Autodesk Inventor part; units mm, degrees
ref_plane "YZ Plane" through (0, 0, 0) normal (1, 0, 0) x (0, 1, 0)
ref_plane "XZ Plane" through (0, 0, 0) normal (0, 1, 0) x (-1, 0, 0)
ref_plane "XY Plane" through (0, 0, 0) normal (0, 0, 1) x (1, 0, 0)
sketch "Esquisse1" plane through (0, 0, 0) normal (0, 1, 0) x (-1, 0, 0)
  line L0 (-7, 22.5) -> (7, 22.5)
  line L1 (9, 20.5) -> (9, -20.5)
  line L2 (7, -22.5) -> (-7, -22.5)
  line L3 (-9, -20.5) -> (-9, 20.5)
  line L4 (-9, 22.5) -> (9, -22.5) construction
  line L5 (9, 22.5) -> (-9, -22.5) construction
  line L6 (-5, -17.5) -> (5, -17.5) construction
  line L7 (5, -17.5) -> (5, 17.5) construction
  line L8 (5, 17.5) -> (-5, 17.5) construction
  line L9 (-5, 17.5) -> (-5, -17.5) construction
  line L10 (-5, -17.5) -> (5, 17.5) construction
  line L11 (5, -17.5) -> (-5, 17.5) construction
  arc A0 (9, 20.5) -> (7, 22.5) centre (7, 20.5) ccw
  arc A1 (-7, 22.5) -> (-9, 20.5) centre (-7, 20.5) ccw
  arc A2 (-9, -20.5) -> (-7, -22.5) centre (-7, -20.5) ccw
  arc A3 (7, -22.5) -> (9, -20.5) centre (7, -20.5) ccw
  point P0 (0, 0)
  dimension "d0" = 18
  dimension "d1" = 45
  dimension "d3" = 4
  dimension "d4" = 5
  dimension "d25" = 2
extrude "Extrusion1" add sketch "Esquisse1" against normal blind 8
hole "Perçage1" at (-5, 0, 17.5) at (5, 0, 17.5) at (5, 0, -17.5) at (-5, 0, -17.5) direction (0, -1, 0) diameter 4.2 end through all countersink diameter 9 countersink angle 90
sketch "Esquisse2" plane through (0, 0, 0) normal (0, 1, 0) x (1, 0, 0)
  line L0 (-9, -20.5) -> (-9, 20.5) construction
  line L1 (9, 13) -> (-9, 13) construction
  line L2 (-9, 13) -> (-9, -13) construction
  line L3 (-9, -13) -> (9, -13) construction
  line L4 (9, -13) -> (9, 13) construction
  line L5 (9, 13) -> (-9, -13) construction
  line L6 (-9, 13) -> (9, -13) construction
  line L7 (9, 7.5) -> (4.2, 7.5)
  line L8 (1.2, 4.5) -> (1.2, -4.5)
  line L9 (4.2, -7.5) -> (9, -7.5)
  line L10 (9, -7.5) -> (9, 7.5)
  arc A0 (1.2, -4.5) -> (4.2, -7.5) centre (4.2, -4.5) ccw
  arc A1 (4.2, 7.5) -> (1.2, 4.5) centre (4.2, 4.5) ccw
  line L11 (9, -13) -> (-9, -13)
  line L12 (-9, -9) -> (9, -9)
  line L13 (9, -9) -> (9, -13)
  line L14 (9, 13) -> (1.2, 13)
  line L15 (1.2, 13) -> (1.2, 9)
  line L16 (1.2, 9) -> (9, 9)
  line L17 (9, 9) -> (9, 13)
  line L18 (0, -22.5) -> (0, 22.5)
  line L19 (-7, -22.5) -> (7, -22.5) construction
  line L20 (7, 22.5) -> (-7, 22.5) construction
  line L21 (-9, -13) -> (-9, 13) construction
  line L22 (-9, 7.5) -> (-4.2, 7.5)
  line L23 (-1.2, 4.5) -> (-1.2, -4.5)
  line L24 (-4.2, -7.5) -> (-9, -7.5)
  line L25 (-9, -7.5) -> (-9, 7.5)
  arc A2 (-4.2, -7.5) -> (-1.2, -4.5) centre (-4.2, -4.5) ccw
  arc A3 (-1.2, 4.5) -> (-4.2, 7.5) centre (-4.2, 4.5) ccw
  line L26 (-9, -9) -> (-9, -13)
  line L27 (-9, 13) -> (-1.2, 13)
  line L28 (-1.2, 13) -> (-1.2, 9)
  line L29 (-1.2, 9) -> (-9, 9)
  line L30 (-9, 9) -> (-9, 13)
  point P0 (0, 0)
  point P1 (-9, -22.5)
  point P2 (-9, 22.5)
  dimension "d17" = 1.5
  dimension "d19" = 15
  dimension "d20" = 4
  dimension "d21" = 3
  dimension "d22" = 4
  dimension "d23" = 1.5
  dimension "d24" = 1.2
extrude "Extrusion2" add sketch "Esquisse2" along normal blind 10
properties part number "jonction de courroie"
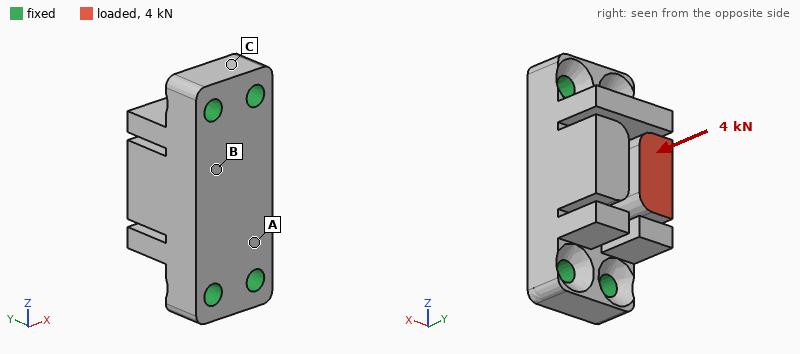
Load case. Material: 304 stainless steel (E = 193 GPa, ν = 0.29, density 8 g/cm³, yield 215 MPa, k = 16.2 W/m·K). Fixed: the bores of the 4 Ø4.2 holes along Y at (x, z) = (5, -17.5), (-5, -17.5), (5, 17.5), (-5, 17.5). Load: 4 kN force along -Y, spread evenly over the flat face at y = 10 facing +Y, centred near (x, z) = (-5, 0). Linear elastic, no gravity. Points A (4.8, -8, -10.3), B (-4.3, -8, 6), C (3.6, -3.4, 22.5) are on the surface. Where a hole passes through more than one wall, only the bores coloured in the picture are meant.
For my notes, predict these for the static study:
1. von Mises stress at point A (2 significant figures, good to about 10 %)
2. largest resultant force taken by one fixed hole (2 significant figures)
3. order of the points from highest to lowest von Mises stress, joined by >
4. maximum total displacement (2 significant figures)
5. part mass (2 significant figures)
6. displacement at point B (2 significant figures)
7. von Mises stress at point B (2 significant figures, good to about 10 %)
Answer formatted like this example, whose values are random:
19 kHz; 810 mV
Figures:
26 MPa; 1.9 kN; B > A > C; 14 µm; 75 g; 7.1 µm; 47 MPa
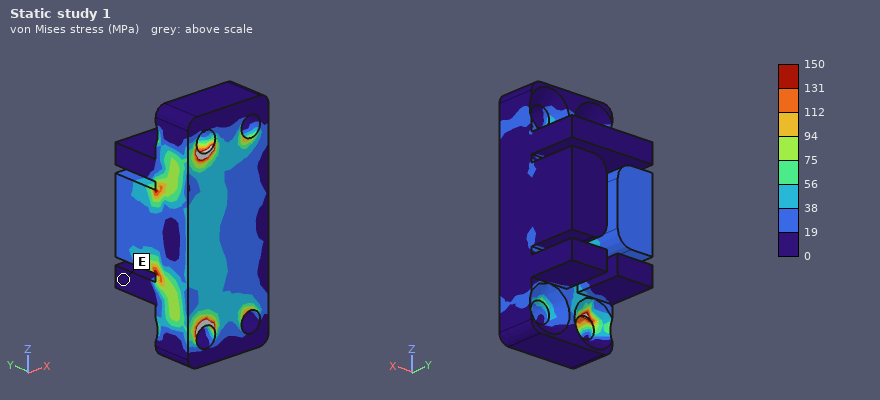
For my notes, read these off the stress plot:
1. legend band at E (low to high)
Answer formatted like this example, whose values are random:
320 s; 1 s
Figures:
0 to 19 MPa
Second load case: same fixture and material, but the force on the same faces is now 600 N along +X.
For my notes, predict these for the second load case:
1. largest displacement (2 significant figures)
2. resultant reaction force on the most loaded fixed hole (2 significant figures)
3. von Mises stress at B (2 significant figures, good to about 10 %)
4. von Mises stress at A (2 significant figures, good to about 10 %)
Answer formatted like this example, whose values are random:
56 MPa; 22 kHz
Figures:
9.5 µm; 450 N; 14 MPa; 5.5 MPa
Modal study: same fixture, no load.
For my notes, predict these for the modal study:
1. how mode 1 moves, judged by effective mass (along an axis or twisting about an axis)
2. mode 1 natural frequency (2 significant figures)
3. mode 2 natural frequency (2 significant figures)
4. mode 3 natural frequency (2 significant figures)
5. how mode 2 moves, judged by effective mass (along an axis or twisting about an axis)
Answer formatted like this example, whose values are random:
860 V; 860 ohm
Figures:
along X; 15 kHz; 17 kHz; 22 kHz; along Y
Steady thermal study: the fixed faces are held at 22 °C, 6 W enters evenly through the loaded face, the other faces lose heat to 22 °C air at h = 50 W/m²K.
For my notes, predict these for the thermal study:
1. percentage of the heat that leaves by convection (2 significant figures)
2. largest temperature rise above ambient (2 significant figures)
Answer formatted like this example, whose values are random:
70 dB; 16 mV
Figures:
29 %; 50 K
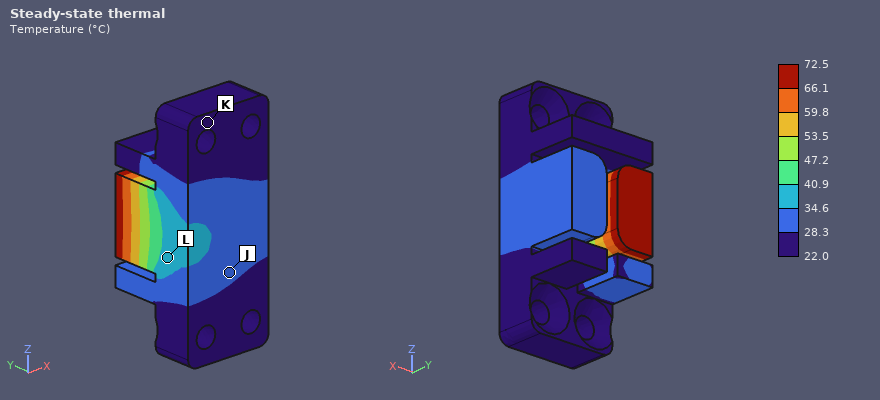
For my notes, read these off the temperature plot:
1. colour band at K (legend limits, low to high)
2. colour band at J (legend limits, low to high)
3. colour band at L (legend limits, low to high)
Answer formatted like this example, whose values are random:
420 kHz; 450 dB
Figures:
22.0 to 28.3 °C; 28.3 to 34.6 °C; 34.6 to 40.9 °C
